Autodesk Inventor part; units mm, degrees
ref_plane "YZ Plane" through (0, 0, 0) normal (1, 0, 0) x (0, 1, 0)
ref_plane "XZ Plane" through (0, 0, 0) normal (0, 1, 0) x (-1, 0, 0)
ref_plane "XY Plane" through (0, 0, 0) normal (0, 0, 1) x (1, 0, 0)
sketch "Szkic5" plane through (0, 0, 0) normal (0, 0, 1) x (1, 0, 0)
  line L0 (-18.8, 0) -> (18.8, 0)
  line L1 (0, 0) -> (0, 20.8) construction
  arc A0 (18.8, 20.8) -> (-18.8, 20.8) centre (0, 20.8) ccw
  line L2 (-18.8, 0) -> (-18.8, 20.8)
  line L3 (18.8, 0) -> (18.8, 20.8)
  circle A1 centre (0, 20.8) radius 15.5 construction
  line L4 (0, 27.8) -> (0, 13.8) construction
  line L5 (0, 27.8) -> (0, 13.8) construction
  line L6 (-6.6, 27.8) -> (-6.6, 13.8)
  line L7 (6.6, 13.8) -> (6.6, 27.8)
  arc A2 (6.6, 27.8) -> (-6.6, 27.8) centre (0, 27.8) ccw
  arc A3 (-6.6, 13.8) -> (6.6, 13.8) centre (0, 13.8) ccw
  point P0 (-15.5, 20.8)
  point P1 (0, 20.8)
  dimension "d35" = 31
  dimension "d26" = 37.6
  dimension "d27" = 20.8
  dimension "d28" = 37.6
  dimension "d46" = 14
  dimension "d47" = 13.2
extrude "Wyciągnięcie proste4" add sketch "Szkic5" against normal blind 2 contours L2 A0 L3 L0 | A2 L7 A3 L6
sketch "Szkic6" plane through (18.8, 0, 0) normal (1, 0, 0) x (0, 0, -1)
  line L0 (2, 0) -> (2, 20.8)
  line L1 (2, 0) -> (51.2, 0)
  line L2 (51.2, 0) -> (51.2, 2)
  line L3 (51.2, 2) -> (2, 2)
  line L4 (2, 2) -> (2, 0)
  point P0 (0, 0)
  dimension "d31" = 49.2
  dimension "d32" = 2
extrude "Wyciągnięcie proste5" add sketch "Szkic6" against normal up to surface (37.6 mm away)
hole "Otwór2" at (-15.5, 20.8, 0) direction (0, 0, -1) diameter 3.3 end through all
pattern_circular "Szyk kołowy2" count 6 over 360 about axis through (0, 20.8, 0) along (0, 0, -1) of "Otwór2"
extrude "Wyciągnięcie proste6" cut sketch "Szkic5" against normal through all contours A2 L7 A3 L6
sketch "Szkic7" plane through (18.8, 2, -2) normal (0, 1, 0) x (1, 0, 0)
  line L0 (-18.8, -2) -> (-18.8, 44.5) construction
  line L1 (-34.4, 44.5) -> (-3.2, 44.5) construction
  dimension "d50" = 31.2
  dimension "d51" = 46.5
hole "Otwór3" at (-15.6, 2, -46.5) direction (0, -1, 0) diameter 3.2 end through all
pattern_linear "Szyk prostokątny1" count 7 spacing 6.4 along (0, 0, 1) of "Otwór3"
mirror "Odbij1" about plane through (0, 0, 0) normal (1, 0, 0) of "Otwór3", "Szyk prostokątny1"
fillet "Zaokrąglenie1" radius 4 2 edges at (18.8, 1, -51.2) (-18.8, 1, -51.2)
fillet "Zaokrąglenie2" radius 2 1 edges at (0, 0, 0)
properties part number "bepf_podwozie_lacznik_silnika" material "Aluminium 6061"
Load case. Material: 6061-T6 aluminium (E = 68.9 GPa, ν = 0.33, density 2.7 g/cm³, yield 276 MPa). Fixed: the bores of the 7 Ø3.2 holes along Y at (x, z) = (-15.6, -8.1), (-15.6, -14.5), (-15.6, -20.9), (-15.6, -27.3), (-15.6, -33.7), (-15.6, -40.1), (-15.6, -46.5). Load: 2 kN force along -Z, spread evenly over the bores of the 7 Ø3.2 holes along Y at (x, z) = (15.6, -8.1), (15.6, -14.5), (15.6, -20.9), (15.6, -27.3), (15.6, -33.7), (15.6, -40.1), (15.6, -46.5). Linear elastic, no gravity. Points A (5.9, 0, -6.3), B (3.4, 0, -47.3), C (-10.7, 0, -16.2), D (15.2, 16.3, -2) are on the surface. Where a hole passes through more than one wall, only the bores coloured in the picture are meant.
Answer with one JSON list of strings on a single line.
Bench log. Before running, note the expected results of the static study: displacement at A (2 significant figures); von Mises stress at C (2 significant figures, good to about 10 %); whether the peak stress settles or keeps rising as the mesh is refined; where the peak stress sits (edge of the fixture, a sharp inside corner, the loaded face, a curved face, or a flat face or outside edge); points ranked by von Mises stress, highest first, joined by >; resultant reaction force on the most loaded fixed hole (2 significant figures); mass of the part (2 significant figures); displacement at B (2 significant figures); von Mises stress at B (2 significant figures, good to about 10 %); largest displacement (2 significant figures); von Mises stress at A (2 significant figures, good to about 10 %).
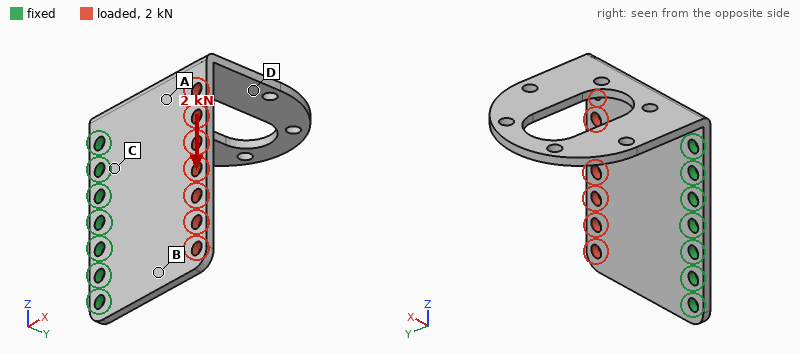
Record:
["32 µm", "57 MPa", "keeps rising", "edge of the fixture", "C > B > A > D", "1.3 kN", "14 g", "28 µm", "30 MPa", "55 µm", "23 MPa"]
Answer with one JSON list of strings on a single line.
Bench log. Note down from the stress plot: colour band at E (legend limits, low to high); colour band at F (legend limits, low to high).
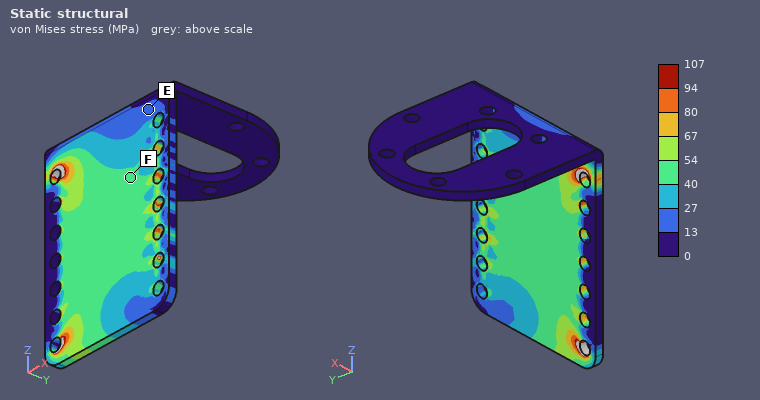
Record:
["13 to 27 MPa", "40 to 54 MPa"]
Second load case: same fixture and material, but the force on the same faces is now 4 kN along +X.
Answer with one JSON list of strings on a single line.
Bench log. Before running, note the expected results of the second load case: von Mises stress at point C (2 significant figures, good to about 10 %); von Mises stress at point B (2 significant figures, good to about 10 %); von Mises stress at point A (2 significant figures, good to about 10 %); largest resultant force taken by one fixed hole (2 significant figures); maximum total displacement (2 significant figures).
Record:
["40 MPa", "37 MPa", "29 MPa", "760 N", "22 µm"]
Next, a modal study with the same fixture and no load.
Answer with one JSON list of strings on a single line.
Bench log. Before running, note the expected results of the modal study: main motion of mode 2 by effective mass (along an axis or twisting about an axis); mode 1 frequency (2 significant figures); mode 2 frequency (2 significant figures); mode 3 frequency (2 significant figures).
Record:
["along Y", "910 Hz", "1200 Hz", "2200 Hz"]
